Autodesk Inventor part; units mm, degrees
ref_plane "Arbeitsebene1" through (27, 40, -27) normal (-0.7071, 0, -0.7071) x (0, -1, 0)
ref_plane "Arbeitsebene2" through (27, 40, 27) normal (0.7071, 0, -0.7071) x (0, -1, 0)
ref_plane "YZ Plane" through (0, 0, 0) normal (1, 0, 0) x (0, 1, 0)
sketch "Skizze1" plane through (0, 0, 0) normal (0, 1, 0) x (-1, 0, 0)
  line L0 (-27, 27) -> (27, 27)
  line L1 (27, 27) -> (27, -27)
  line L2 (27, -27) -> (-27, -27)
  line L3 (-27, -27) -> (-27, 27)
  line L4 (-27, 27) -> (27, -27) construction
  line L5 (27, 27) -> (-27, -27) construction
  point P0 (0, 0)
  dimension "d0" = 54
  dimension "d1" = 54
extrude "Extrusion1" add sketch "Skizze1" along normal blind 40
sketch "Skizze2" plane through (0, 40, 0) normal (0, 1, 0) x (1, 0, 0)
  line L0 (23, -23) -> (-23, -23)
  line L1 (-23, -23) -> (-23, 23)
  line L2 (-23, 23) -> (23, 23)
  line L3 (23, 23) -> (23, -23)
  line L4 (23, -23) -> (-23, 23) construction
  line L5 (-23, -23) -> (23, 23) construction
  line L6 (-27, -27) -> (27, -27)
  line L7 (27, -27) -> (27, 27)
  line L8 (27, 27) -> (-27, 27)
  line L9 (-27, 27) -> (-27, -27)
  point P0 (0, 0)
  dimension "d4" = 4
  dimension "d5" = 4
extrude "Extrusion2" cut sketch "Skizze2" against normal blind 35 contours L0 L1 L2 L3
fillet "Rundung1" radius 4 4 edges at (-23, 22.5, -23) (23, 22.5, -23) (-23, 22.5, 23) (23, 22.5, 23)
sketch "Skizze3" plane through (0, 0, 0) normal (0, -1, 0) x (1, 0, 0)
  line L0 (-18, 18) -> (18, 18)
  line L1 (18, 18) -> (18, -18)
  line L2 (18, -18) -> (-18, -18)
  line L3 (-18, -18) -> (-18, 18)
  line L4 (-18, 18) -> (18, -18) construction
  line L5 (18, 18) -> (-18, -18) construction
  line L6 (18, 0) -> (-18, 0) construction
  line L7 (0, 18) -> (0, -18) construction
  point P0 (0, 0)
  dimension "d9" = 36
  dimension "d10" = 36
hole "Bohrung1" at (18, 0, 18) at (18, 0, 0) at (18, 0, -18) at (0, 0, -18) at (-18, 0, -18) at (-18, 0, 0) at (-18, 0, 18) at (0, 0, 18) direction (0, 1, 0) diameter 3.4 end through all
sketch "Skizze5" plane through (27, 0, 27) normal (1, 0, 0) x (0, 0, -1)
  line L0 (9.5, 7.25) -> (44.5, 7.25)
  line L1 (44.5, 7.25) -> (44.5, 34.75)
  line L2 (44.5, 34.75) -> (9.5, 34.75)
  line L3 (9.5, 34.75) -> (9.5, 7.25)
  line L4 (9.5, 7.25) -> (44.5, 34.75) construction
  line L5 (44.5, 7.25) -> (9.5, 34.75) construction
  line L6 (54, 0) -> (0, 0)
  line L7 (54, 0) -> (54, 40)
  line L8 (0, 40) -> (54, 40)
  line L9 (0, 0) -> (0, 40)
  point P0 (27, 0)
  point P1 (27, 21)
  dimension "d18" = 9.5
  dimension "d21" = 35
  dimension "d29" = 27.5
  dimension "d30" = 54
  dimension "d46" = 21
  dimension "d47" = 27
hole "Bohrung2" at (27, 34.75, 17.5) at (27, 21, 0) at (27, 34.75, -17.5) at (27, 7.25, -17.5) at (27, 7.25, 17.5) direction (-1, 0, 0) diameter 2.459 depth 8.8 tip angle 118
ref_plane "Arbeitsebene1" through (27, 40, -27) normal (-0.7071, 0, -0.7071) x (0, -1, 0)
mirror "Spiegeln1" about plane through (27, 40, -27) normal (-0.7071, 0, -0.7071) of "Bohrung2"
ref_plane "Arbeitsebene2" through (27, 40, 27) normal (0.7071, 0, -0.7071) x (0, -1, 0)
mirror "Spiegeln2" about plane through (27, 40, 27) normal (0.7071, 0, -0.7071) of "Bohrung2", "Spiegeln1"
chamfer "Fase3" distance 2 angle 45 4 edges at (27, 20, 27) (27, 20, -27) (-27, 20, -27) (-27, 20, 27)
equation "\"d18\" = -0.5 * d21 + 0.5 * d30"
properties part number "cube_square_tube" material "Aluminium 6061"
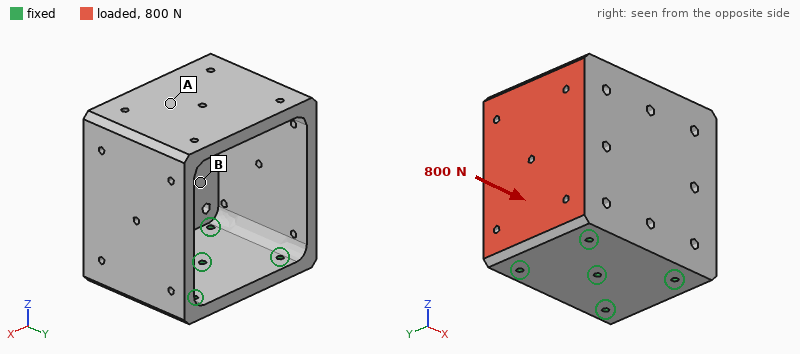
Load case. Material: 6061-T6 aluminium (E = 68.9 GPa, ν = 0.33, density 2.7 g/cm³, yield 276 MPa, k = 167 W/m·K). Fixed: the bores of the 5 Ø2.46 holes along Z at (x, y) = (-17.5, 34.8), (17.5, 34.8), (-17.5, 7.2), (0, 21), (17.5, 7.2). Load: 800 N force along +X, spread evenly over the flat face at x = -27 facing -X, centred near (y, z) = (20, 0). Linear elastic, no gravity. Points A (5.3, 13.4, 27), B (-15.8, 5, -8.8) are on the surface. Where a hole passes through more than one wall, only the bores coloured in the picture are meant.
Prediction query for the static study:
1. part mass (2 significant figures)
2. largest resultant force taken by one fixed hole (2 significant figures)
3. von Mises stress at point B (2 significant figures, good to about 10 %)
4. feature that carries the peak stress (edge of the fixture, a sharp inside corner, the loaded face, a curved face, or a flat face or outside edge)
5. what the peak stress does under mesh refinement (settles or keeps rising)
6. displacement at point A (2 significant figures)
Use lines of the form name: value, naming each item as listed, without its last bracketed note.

part mass: 110 g
largest resultant force taken by one fixed hole: 740 N
von Mises stress at point B: 7.5 MPa
feature that carries the peak stress: edge of the fixture
what the peak stress does under mesh refinement: keeps rising
displacement at point A: 27 µm
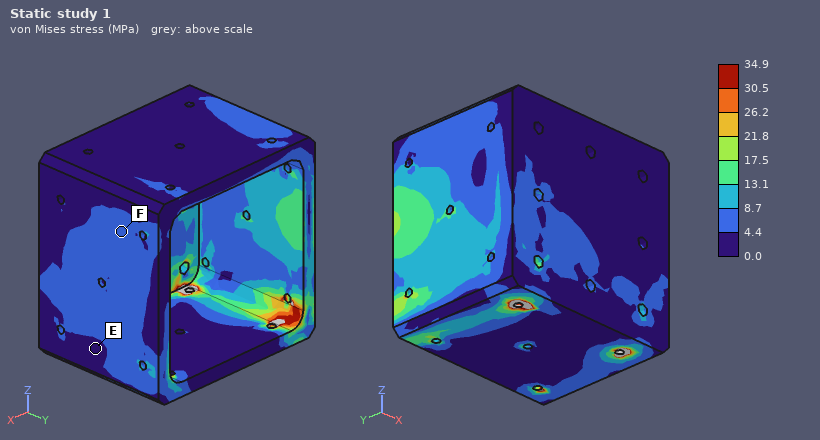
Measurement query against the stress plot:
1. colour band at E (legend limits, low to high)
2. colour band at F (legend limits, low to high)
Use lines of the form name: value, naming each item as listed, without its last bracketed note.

colour band at E: 0.0 to 4.4 MPa
colour band at F: 4.4 to 8.7 MPa
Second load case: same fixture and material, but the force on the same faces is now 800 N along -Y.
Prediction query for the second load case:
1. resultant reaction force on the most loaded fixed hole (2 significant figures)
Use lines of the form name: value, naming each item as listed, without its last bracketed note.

resultant reaction force on the most loaded fixed hole: 760 N
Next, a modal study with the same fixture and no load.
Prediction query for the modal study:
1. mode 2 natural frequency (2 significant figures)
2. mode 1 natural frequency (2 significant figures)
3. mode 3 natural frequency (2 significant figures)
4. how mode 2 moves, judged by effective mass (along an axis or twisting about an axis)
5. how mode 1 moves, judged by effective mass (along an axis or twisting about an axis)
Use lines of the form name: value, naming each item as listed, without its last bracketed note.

mode 2 natural frequency: 3000 Hz
mode 1 natural frequency: 2600 Hz
mode 3 natural frequency: 6000 Hz
how mode 2 moves, judged by effective mass: along Y
how mode 1 moves, judged by effective mass: along X
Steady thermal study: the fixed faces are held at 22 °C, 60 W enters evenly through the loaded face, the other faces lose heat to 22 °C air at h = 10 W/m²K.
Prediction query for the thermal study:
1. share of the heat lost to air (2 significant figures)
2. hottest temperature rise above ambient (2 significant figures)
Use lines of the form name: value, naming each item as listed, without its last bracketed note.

share of the heat lost to air: 4.6 %
hottest temperature rise above ambient: 34 K
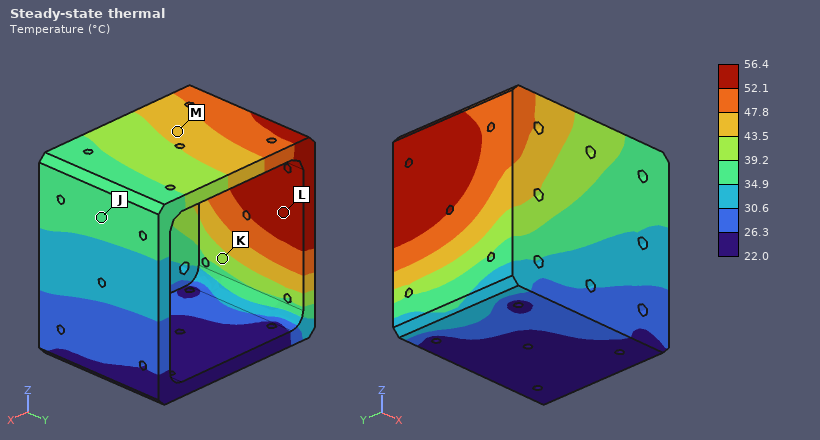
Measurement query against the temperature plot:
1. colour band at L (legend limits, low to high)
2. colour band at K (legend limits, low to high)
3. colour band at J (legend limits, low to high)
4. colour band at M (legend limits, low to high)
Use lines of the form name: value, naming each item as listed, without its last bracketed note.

colour band at L: 52.1 to 56.4 °C
colour band at K: 39.2 to 43.5 °C
colour band at J: 34.9 to 39.2 °C
colour band at M: 43.5 to 47.8 °C
